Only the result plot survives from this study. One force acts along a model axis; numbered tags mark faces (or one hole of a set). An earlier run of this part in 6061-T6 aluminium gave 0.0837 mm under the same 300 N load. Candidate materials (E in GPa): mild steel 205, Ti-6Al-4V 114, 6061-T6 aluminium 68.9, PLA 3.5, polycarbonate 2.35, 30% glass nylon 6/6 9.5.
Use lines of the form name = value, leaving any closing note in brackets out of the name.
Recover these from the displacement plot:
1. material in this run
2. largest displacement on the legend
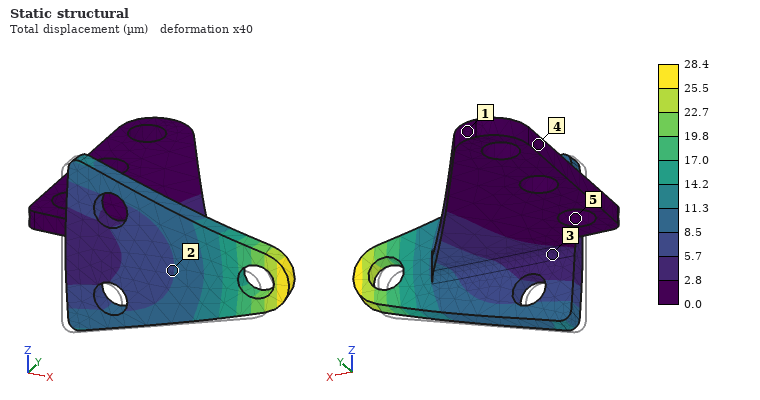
material in this run = mild steel
largest displacement on the legend = 28.4 µm
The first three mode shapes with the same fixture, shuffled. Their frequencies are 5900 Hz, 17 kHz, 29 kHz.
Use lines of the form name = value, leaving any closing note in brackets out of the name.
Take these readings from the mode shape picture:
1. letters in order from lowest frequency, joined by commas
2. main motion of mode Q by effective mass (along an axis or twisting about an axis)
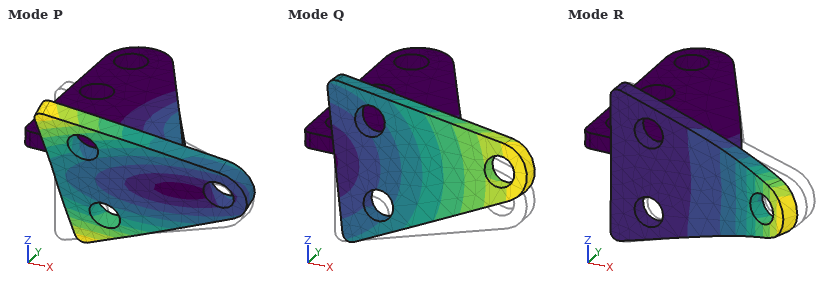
letters in order from lowest frequency, joined by commas = Q, P, R
main motion of mode Q by effective mass = along Z
